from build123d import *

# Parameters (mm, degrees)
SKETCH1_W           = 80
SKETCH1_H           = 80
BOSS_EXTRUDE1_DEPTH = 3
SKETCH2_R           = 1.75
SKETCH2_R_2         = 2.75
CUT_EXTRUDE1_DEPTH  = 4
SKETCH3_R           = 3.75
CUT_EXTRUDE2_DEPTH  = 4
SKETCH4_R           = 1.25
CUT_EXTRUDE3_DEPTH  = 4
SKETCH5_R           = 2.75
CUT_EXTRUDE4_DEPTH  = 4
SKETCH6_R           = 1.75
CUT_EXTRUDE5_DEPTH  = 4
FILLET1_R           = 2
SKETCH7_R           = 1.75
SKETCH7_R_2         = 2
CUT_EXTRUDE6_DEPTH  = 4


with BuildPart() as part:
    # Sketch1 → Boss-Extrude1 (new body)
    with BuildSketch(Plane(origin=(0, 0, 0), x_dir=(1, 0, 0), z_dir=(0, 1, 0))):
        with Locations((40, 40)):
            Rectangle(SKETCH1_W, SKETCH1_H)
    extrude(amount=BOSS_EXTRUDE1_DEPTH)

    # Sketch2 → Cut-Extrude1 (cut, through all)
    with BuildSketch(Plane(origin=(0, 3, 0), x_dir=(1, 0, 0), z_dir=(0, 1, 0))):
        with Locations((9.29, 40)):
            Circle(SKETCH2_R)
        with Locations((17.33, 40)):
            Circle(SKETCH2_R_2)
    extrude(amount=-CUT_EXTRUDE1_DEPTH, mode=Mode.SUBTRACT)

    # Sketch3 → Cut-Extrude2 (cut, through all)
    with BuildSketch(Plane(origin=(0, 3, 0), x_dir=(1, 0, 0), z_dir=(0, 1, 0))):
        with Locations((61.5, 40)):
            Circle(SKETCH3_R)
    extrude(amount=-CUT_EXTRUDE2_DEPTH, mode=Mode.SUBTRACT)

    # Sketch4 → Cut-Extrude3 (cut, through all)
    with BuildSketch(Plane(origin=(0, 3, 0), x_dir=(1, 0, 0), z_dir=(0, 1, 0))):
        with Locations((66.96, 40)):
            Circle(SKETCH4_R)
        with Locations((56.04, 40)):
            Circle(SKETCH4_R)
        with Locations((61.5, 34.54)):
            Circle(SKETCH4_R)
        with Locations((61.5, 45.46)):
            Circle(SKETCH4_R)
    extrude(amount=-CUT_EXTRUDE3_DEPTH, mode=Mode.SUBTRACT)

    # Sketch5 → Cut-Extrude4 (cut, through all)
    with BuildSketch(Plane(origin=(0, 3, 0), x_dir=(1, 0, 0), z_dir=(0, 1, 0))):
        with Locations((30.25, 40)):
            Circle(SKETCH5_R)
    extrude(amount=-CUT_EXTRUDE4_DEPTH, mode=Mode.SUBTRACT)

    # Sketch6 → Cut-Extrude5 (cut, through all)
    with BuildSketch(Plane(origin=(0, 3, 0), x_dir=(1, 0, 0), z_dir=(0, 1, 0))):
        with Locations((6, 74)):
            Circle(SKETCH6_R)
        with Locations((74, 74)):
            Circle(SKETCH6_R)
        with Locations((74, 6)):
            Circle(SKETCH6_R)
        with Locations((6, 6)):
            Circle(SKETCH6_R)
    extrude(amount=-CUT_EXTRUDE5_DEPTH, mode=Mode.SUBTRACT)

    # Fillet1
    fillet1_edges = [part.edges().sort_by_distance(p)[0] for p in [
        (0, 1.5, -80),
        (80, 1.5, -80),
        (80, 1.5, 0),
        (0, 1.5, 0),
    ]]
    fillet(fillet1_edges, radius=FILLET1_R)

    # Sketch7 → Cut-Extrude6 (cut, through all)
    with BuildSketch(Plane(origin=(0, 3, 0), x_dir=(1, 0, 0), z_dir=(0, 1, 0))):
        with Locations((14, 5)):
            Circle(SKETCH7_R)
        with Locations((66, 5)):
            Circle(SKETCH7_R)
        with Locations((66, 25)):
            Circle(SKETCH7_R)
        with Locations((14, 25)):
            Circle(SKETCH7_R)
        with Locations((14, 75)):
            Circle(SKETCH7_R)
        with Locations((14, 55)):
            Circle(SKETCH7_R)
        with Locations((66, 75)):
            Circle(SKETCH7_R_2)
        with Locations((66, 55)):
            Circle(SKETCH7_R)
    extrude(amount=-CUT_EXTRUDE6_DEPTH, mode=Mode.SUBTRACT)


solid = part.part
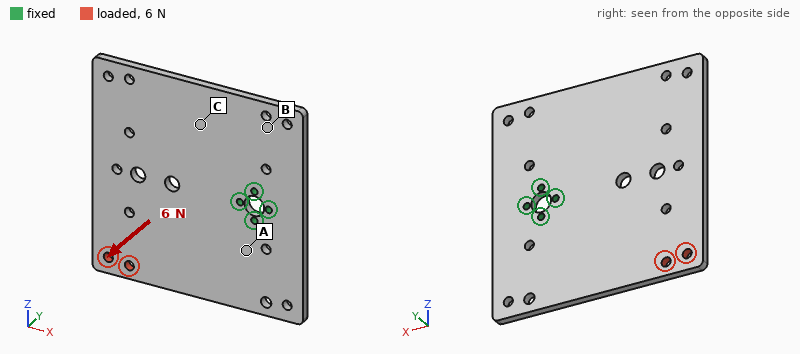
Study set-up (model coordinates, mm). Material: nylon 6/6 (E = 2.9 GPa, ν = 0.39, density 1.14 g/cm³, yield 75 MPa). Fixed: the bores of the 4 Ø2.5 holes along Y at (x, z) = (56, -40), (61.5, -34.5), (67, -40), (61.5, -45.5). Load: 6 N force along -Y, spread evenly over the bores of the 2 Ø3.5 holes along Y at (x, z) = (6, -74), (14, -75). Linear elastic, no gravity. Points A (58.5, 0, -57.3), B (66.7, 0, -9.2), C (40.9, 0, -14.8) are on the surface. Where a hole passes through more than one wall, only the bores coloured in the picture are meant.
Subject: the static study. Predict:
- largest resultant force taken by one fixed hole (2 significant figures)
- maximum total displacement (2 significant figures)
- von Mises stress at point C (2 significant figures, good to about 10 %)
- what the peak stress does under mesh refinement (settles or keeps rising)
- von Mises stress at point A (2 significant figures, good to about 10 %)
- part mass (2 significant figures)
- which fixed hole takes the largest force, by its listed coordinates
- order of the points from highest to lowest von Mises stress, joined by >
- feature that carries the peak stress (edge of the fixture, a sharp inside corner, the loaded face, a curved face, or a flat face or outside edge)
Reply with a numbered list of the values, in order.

1. 18 N
2. 1.3 mm
3. 1.3 MPa
4. keeps rising
5. 2.5 MPa
6. 21 g
7. (56, -40)
8. A > C > B
9. edge of the fixture
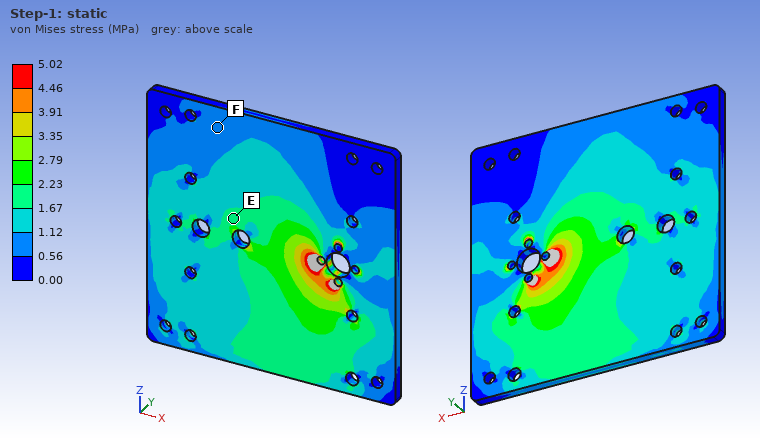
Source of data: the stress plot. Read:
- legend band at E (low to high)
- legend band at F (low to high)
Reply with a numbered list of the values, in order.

1. 1.67 to 2.23 MPa
2. 0.56 to 1.12 MPa
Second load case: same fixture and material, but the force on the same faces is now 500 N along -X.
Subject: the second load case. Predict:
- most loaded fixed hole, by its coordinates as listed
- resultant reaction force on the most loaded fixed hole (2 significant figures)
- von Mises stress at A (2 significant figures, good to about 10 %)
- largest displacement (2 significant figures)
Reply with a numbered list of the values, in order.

1. (61.5, -45.5)
2. 880 N
3. 8.9 MPa
4. 1.1 mm
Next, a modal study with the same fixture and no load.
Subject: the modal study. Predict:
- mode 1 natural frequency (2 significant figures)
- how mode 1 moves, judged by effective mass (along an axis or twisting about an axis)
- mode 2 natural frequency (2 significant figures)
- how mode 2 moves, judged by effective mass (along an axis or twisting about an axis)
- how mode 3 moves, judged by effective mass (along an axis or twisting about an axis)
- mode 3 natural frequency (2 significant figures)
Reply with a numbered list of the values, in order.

1. 210 Hz
2. along Y
3. 280 Hz
4. twisting about X
5. along Y
6. 610 Hz
